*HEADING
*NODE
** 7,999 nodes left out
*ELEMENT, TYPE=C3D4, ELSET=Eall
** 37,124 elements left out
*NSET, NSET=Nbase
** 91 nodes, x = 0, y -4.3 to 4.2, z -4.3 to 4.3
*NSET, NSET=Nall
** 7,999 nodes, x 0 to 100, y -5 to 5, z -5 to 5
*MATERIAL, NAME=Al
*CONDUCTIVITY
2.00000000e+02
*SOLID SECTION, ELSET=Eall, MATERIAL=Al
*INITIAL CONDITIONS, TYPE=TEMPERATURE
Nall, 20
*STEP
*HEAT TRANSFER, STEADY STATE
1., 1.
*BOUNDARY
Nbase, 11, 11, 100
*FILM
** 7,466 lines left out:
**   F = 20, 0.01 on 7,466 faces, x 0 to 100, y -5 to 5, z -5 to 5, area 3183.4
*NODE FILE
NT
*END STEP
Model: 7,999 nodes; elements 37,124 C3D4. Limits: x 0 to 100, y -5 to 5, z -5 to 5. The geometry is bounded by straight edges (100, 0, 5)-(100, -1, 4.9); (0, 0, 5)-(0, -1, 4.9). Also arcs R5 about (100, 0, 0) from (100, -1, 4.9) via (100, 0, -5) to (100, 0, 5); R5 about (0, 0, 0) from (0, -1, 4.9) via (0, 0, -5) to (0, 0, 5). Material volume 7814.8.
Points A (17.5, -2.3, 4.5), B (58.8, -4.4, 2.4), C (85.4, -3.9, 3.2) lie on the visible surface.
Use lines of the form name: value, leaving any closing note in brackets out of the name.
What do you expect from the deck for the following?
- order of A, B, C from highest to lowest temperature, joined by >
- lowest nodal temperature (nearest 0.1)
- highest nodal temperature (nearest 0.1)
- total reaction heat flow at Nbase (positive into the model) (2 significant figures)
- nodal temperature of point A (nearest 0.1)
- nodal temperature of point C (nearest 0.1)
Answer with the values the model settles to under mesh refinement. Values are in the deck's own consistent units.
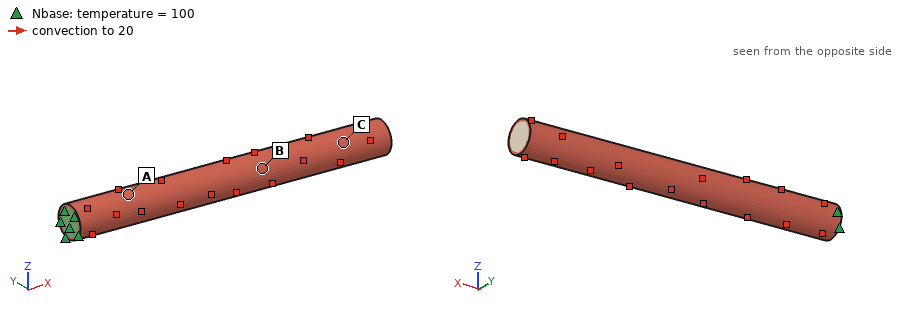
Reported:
order of A, B, C from highest to lowest temperature, joined by >: A > B > C
lowest nodal temperature: 92.5
highest nodal temperature: 100.0
total reaction heat flow at Nbase (positive into the model): 2400
nodal temperature of point A: 97.6
nodal temperature of point C: 92.6
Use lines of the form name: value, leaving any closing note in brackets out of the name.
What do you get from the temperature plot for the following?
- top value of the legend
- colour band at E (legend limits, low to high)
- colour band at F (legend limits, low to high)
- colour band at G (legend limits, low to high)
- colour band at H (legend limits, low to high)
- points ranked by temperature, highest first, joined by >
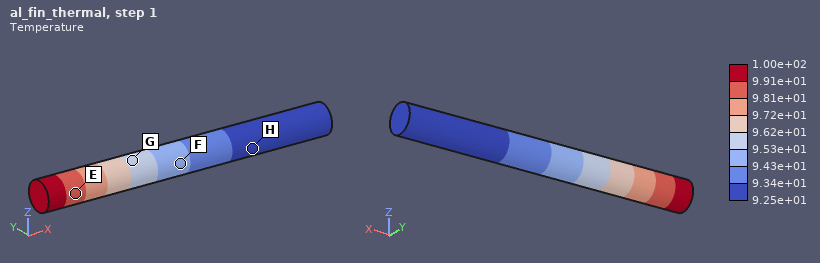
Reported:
top value of the legend: 1.00e+02
colour band at E: 9.81e+01 to 9.91e+01
colour band at F: 9.43e+01 to 9.53e+01
colour band at G: 9.53e+01 to 9.62e+01
colour band at H: 9.25e+01 to 9.34e+01
points ranked by temperature, highest first, joined by >: E > G > F > H
